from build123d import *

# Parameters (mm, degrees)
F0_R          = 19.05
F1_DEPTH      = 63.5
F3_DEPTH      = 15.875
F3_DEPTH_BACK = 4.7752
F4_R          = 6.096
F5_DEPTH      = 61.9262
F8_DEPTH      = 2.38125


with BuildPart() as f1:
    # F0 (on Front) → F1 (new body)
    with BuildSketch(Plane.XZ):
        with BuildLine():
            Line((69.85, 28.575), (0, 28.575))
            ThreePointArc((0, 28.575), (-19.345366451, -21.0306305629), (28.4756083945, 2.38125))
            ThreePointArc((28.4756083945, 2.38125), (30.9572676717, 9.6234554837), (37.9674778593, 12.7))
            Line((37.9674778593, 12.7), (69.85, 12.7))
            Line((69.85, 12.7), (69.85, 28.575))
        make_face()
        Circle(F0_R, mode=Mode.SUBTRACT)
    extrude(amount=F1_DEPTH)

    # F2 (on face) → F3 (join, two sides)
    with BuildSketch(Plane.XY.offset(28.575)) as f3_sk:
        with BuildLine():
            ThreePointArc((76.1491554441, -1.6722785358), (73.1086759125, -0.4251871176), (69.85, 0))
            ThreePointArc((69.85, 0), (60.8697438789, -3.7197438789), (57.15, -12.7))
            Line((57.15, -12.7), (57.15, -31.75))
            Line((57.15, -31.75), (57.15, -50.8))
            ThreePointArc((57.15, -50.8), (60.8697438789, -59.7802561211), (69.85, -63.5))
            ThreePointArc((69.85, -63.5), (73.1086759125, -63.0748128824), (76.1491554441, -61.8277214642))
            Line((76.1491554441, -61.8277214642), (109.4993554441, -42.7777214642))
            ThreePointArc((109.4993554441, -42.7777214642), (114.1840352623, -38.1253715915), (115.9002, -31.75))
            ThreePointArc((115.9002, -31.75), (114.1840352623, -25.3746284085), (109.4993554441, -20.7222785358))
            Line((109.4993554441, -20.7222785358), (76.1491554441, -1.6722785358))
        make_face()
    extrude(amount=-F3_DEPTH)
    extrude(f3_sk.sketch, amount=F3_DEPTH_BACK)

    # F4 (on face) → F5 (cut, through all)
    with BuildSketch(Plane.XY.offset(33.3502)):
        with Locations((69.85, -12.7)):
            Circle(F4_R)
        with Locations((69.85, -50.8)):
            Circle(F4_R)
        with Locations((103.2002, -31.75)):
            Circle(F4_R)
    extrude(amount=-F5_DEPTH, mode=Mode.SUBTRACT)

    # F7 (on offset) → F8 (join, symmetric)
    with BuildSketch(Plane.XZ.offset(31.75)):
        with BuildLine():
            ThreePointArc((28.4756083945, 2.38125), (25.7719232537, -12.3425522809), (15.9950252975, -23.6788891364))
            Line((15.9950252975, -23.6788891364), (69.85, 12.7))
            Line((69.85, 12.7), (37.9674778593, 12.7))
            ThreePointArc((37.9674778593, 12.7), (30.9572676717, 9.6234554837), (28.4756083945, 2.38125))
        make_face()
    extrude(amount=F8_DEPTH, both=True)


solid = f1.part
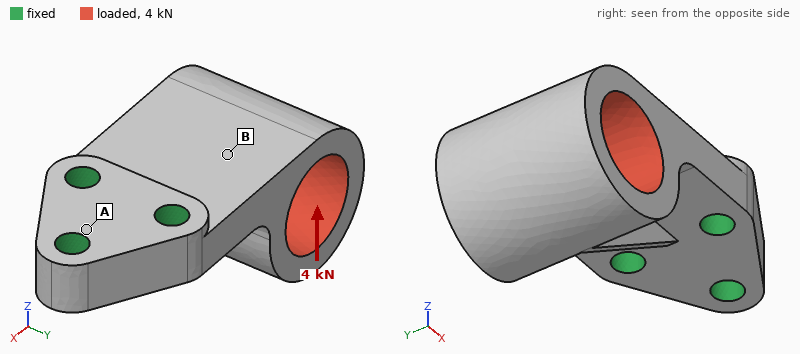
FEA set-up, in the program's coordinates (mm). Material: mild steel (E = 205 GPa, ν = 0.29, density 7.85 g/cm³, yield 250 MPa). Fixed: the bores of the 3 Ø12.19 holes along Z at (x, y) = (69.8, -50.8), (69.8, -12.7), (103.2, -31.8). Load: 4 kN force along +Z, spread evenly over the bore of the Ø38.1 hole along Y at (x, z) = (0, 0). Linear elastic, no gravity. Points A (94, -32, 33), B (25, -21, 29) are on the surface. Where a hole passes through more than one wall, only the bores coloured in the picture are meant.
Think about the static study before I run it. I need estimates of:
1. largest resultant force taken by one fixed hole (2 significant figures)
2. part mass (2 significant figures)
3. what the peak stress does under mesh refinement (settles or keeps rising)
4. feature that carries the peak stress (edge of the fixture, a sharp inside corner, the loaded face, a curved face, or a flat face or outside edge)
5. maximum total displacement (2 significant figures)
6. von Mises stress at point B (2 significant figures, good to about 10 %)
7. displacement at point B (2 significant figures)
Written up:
2.5 kN
1.4 kg
keeps rising
edge of the fixture
0.11 mm
17 MPa
0.034 mm
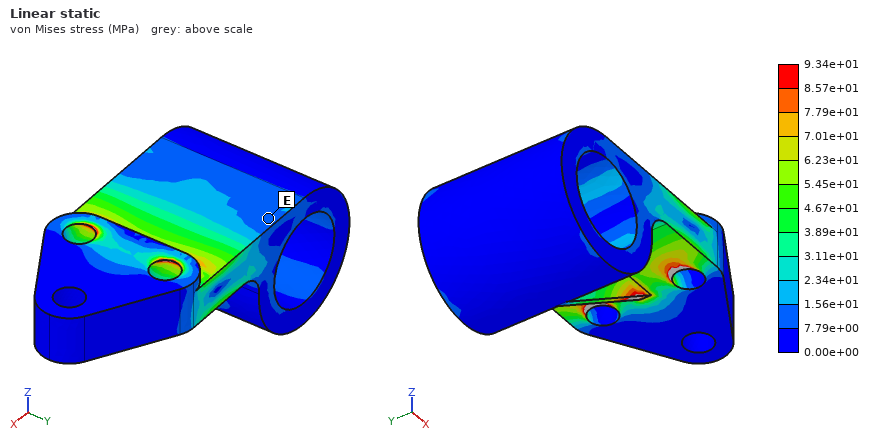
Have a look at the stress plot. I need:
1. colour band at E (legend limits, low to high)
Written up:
7.79e+00 to 1.56e+01 MPa
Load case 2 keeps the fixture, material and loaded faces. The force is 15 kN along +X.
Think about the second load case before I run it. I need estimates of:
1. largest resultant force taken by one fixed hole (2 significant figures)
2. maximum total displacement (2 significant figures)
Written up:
7.0 kN
0.17 mm
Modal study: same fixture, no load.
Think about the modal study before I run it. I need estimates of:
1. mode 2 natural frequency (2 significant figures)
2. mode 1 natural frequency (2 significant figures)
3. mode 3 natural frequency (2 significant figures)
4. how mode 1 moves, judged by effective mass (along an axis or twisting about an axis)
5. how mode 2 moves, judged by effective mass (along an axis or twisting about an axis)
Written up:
2600 Hz
1200 Hz
4400 Hz
along Z
along Y
